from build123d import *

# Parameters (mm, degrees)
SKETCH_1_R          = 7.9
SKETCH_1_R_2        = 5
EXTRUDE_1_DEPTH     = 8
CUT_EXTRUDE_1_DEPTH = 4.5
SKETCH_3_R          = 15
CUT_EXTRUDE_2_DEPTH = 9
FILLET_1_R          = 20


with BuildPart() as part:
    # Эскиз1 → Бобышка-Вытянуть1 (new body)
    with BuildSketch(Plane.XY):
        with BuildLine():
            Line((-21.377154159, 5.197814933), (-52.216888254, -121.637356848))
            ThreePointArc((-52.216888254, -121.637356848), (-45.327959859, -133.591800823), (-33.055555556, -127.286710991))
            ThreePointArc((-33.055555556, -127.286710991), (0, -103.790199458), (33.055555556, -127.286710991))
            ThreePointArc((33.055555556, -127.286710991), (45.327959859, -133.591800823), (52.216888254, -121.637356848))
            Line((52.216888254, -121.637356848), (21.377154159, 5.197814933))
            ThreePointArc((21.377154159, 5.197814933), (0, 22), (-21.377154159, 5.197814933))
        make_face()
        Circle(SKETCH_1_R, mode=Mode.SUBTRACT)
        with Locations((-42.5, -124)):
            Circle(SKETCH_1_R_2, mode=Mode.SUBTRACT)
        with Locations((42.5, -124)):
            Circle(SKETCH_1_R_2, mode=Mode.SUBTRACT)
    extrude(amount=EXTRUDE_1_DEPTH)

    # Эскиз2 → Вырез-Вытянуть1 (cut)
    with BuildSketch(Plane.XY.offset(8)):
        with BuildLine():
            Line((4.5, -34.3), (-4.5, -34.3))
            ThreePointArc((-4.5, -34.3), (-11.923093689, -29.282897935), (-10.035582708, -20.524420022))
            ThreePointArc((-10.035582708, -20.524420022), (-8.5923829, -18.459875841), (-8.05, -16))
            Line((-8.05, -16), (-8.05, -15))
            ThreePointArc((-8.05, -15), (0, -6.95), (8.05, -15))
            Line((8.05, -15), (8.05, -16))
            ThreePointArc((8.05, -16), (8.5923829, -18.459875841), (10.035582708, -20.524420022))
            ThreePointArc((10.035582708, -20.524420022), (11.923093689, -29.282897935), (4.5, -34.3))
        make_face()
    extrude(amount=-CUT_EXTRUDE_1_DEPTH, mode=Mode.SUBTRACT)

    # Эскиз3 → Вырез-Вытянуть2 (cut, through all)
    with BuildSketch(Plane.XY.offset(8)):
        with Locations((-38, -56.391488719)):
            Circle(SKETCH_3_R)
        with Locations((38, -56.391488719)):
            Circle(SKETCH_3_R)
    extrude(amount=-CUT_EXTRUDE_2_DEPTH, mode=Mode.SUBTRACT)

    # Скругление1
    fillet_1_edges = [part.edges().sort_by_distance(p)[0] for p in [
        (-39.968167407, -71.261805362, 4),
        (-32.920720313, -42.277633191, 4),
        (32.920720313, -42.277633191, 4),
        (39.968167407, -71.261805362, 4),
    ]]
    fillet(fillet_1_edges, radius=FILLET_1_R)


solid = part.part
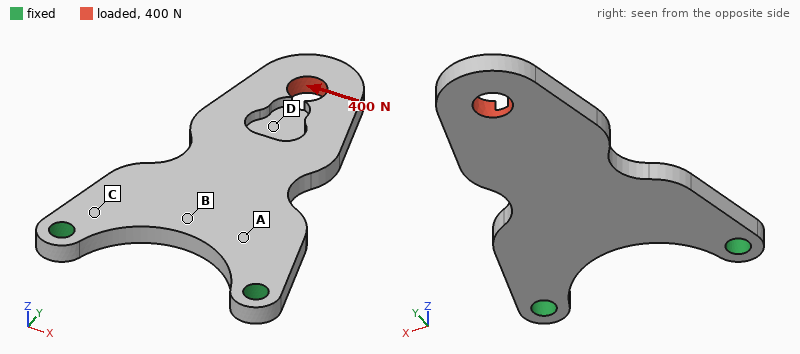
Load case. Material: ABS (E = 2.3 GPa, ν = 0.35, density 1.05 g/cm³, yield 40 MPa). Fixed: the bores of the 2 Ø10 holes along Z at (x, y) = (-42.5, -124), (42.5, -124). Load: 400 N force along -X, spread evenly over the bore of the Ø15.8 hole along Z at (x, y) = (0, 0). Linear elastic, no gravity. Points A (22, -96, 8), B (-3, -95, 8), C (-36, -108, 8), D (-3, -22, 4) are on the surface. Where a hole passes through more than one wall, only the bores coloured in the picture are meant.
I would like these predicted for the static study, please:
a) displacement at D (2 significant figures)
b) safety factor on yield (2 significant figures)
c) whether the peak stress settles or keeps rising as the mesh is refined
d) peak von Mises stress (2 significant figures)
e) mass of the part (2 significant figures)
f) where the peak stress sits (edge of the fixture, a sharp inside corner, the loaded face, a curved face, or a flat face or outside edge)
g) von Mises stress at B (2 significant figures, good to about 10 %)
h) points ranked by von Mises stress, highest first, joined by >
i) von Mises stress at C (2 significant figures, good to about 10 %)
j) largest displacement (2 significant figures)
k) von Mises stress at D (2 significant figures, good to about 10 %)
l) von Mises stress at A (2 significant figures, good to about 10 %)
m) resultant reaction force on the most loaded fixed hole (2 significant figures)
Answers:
0.42 mm
3.1
settles
13 MPa
69 g
a curved face
1.1 MPa
D > C > A > B
3.6 MPa
0.86 mm
5.3 MPa
2.3 MPa
610 N
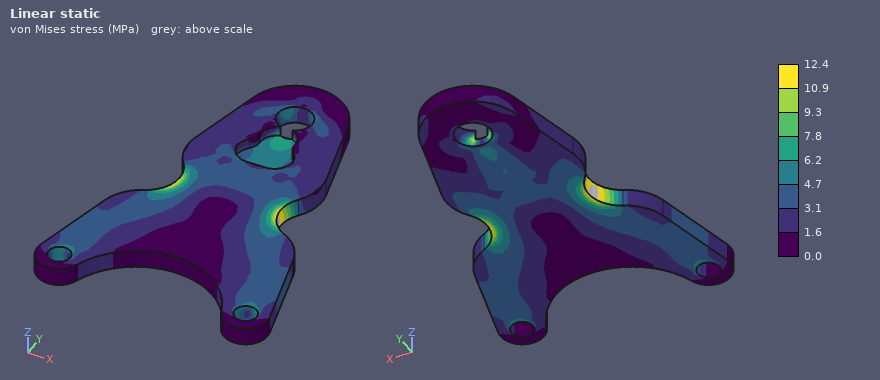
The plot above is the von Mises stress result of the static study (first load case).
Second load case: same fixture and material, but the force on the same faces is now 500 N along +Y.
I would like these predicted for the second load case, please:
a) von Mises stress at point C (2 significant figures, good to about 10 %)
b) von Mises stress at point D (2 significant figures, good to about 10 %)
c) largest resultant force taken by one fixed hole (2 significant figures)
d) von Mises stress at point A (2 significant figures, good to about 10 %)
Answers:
1.4 MPa
2.6 MPa
280 N
1.2 MPa
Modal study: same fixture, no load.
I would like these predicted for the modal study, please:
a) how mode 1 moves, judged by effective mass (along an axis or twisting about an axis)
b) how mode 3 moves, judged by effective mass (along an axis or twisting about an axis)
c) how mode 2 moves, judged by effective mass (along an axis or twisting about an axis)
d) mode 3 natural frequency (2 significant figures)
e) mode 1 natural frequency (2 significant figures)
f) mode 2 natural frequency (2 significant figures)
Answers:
along Z
twisting about Y
along Z
590 Hz
110 Hz
550 Hz
